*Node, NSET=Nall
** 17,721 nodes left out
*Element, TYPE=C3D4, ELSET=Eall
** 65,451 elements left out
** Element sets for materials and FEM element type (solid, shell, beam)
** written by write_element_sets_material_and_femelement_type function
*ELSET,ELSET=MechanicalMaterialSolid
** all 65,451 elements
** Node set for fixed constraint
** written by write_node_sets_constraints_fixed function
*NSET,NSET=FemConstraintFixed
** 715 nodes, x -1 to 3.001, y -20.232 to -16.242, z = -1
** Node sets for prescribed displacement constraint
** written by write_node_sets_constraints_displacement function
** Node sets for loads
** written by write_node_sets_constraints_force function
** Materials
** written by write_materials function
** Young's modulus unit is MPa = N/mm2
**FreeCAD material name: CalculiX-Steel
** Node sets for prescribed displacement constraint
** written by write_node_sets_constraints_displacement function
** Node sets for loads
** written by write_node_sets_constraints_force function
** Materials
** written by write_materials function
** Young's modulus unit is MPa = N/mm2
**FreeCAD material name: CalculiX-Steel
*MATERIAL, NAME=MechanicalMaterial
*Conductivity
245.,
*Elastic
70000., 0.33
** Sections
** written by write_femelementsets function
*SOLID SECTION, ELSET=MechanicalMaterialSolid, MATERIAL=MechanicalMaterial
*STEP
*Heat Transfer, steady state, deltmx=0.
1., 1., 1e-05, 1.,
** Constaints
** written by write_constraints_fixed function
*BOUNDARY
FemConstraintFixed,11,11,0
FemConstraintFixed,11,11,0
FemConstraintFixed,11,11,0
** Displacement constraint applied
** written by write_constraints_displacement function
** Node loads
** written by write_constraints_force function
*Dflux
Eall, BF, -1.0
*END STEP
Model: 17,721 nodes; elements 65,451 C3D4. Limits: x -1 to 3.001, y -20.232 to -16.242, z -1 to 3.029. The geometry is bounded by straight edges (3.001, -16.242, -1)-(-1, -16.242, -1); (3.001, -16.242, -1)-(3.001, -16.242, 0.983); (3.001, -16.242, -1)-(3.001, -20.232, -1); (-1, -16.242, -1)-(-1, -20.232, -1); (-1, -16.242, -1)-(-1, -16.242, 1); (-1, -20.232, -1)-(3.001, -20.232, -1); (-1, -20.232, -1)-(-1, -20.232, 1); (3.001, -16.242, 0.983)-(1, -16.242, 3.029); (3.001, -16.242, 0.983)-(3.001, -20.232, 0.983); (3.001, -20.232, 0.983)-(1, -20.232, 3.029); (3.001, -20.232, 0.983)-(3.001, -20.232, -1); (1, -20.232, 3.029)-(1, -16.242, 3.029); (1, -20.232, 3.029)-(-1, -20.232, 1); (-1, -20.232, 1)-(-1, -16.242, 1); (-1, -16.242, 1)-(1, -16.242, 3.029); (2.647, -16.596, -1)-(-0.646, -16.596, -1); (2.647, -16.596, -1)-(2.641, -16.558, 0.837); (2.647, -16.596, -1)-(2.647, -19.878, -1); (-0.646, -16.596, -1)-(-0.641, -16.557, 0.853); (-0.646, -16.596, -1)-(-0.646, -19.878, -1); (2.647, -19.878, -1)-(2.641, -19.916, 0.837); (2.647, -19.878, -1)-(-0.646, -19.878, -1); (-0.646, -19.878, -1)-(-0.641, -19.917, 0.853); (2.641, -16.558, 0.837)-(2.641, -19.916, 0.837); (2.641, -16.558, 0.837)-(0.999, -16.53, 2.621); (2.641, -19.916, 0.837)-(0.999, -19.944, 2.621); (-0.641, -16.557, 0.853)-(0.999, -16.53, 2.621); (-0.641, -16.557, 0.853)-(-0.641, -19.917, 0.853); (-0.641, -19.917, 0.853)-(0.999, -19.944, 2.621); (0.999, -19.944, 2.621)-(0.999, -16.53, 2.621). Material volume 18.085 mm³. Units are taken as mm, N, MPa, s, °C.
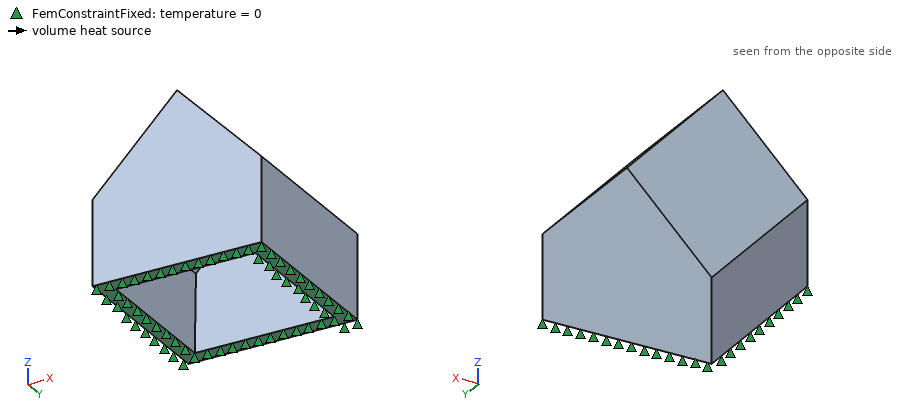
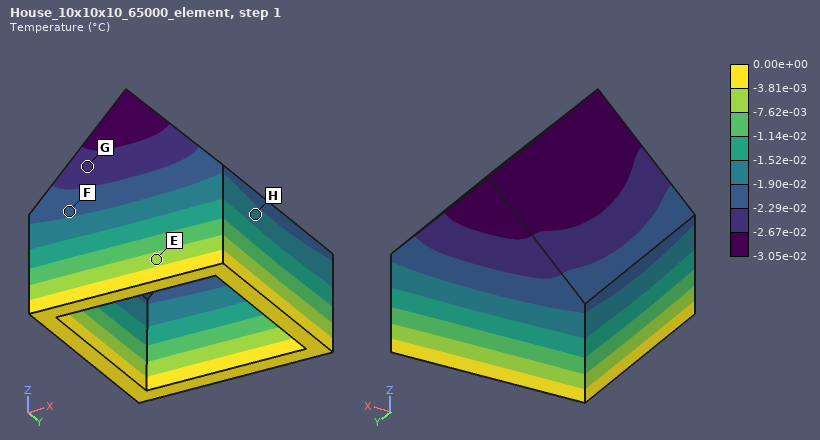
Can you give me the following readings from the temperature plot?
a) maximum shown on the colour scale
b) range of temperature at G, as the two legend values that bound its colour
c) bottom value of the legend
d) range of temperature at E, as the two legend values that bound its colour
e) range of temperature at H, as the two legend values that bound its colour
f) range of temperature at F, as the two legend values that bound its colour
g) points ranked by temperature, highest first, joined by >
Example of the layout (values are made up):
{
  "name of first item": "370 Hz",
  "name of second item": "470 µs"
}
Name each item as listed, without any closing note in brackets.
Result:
{
  "maximum shown on the colour scale": "0.00e+00 °C",
  "range of temperature at G, as the two legend values that bound its colour": "-2.67e-02 to -2.29e-02 °C",
  "bottom value of the legend": "-3.05e-02 °C",
  "range of temperature at E, as the two legend values that bound its colour": "-7.62e-03 to -3.81e-03 °C",
  "range of temperature at H, as the two legend values that bound its colour": "-1.90e-02 to -1.52e-02 °C",
  "range of temperature at F, as the two legend values that bound its colour": "-2.29e-02 to -1.90e-02 °C",
  "points ranked by temperature, highest first, joined by >": "E > H > F > G"
}
